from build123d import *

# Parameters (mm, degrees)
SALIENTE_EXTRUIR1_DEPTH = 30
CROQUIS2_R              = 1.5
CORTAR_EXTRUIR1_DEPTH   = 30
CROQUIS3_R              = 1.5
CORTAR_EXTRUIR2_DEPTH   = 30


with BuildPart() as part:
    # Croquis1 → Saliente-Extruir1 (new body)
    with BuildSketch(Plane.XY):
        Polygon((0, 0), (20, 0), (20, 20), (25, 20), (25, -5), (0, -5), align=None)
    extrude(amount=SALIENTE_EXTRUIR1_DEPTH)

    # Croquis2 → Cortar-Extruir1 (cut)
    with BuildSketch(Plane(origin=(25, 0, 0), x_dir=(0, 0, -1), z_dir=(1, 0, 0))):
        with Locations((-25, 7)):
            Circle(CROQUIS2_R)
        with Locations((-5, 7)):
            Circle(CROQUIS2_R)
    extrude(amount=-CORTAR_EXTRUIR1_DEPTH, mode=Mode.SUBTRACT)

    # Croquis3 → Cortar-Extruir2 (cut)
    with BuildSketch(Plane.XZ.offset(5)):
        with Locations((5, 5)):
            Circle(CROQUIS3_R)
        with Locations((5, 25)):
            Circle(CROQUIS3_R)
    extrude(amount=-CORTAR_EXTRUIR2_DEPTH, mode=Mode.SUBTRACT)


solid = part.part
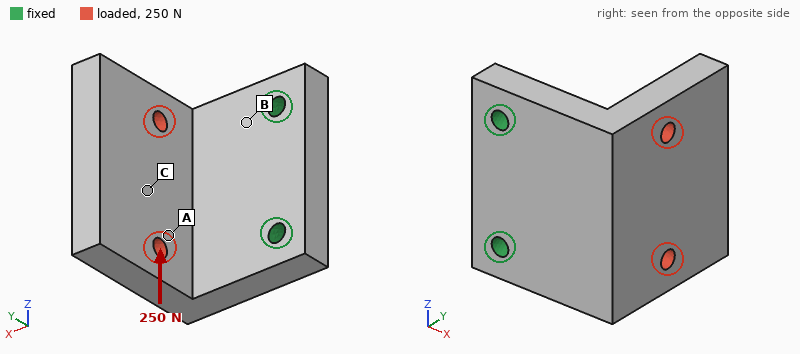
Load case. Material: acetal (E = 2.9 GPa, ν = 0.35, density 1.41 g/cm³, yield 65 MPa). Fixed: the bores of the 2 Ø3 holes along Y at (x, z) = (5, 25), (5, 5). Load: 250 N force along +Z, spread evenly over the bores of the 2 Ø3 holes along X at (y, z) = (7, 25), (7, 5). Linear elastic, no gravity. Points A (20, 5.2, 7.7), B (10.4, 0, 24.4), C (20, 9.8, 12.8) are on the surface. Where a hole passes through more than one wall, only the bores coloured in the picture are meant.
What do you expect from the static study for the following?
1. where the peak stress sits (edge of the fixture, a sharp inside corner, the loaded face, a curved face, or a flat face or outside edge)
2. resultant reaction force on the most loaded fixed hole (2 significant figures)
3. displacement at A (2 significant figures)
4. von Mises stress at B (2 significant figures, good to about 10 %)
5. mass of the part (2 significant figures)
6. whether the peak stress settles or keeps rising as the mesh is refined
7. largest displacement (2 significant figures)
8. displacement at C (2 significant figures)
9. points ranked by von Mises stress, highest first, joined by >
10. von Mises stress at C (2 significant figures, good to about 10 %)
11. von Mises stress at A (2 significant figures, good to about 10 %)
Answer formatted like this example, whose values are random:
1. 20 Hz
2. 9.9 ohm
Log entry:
1. edge of the fixture
2. 260 N
3. 0.21 mm
4. 11 MPa
5. 9.3 g
6. keeps rising
7. 0.48 mm
8. 0.26 mm
9. B > A > C
10. 2.7 MPa
11. 6.5 MPa
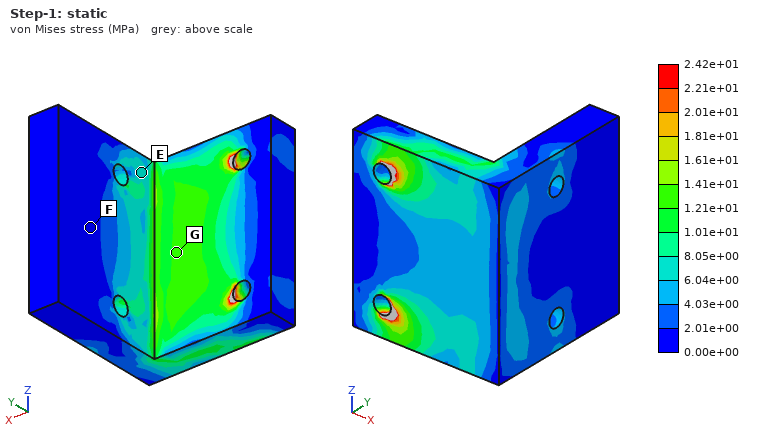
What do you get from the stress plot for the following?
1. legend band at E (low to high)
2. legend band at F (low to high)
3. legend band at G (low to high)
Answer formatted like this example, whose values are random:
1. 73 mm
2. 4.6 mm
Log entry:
1. 6.04e+00 to 8.05e+00 MPa
2. 0.00e+00 to 2.01e+00 MPa
3. 1.21e+01 to 1.41e+01 MPa
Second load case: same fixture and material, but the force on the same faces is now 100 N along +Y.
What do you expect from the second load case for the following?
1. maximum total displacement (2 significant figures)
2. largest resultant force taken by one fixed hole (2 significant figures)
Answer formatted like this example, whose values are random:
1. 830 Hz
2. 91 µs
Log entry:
1. 0.50 mm
2. 50 N
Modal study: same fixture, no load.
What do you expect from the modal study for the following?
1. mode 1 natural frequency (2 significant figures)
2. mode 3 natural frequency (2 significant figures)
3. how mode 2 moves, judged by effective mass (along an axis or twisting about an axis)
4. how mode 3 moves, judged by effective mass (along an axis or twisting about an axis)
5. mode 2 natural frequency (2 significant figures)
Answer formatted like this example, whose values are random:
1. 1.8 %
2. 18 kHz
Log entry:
1. 940 Hz
2. 2600 Hz
3. along Z
4. along Y
5. 1700 Hz
